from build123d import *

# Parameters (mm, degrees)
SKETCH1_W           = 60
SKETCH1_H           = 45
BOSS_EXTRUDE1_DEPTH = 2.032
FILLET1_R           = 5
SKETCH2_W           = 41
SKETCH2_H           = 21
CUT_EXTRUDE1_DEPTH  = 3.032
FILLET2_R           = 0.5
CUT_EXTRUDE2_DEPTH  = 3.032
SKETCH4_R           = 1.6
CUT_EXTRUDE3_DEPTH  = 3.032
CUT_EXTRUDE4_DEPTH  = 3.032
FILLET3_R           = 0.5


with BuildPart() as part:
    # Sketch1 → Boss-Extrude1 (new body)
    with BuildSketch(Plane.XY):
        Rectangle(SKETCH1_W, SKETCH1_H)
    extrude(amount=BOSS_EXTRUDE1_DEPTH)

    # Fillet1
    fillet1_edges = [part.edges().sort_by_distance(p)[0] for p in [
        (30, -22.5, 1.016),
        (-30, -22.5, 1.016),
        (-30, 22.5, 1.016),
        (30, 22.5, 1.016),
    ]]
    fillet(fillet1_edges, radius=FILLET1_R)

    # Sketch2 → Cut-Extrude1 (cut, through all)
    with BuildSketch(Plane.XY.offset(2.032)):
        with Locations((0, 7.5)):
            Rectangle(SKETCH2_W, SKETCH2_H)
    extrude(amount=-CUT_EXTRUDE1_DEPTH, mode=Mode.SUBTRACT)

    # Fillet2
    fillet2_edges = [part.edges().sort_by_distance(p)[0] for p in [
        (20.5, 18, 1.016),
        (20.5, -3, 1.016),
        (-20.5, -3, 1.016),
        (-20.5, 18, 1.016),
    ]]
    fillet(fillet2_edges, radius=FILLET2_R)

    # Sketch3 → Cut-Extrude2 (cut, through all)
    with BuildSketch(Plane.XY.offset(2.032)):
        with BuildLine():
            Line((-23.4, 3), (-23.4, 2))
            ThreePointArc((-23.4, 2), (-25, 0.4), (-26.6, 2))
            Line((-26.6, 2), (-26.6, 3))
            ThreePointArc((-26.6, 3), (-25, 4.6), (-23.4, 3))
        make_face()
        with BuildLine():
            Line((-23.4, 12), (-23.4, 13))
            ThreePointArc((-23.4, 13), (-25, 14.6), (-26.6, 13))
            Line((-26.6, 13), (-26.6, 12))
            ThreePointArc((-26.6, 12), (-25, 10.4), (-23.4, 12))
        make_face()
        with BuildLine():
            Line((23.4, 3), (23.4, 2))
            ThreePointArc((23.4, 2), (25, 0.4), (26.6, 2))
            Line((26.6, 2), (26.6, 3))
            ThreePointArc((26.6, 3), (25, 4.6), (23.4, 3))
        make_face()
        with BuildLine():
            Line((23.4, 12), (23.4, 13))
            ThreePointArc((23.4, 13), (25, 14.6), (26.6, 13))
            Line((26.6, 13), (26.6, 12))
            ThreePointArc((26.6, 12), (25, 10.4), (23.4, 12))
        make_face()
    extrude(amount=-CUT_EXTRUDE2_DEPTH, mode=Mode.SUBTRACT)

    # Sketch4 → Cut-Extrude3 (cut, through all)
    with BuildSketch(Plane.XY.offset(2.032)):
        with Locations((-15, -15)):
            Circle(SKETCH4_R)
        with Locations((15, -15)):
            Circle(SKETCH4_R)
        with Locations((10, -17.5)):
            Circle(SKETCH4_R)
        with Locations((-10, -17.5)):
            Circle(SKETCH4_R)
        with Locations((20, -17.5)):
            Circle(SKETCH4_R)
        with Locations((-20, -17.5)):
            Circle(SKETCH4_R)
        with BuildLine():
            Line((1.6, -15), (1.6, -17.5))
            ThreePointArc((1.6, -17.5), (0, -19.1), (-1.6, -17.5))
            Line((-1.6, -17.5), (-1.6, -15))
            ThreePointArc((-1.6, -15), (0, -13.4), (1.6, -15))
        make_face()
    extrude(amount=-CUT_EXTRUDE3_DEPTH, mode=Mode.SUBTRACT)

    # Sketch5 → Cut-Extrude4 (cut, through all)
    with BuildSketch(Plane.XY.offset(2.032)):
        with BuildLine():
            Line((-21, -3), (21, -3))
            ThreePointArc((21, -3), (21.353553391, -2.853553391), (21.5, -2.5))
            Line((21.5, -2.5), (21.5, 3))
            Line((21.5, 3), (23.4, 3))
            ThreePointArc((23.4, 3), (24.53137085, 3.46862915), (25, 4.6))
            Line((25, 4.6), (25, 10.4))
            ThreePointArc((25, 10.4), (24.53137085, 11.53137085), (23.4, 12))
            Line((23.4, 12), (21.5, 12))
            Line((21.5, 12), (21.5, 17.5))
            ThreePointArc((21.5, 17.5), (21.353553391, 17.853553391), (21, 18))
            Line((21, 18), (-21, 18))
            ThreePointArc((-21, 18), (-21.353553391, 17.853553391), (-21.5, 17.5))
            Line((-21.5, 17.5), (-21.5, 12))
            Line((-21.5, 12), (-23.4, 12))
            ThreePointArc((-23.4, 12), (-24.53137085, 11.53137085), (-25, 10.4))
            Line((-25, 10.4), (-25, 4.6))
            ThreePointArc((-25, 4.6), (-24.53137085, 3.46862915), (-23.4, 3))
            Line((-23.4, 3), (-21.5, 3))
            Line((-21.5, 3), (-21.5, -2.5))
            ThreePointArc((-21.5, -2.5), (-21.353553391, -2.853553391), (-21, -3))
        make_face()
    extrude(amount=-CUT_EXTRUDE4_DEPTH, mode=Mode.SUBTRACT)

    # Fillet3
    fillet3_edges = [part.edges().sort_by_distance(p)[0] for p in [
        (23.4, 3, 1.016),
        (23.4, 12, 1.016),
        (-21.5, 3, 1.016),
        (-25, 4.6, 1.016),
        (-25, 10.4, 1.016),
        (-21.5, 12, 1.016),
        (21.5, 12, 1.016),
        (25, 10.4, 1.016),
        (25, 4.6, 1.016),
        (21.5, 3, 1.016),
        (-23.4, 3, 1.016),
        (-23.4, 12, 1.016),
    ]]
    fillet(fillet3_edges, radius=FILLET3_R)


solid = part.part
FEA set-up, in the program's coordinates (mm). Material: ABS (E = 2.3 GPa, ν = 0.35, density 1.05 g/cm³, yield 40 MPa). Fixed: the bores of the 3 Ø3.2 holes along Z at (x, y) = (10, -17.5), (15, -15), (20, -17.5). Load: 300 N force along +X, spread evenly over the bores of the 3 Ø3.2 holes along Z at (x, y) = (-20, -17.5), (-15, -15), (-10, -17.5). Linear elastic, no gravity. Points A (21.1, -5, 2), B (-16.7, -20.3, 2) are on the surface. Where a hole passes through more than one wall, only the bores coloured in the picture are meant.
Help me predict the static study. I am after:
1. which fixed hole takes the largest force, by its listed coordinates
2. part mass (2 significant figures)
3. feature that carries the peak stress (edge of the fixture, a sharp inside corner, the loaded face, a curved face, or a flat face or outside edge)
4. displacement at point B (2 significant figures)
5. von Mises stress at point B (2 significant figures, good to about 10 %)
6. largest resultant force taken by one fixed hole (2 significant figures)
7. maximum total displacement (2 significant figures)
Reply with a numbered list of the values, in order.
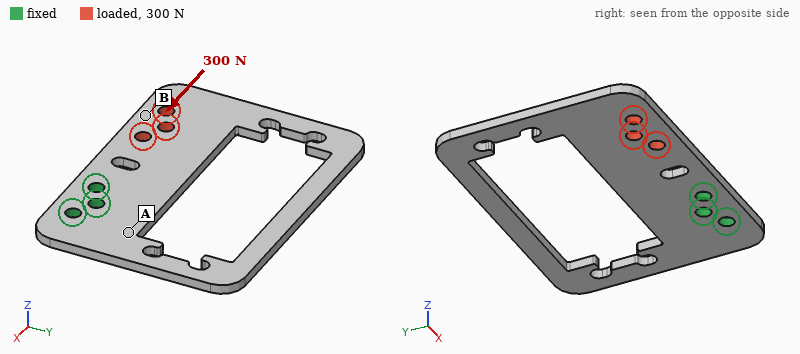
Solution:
1. (10, -17.5)
2. 3.4 g
3. a curved face
4. 0.25 mm
5. 7.6 MPa
6. 210 N
7. 0.36 mm
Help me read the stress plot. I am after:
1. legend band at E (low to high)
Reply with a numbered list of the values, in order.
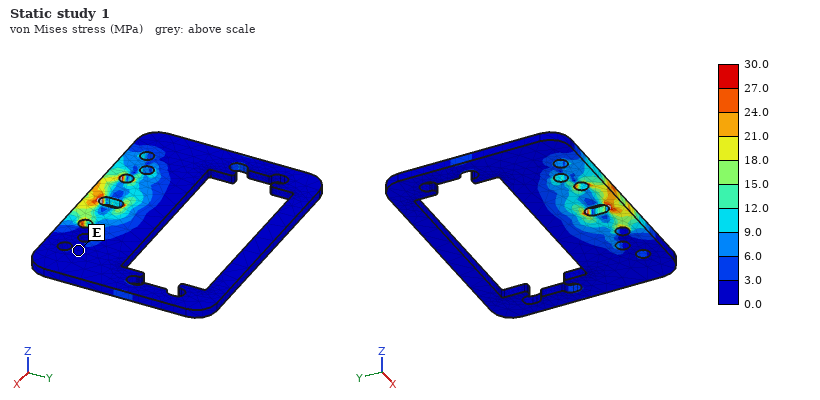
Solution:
1. 0.0 to 3.0 MPa
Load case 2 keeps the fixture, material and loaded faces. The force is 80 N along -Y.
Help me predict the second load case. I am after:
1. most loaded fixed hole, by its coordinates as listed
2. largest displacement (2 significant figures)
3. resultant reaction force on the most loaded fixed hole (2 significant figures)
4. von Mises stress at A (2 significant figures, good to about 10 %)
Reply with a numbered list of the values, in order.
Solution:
1. (10, -17.5)
2. 0.74 mm
3. 220 N
4. 2.9 MPa
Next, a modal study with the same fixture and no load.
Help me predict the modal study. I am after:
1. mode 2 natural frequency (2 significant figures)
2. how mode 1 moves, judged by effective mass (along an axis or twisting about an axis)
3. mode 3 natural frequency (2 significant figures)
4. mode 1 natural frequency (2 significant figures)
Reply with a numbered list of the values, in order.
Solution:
1. 290 Hz
2. along Z
3. 510 Hz
4. 170 Hz
